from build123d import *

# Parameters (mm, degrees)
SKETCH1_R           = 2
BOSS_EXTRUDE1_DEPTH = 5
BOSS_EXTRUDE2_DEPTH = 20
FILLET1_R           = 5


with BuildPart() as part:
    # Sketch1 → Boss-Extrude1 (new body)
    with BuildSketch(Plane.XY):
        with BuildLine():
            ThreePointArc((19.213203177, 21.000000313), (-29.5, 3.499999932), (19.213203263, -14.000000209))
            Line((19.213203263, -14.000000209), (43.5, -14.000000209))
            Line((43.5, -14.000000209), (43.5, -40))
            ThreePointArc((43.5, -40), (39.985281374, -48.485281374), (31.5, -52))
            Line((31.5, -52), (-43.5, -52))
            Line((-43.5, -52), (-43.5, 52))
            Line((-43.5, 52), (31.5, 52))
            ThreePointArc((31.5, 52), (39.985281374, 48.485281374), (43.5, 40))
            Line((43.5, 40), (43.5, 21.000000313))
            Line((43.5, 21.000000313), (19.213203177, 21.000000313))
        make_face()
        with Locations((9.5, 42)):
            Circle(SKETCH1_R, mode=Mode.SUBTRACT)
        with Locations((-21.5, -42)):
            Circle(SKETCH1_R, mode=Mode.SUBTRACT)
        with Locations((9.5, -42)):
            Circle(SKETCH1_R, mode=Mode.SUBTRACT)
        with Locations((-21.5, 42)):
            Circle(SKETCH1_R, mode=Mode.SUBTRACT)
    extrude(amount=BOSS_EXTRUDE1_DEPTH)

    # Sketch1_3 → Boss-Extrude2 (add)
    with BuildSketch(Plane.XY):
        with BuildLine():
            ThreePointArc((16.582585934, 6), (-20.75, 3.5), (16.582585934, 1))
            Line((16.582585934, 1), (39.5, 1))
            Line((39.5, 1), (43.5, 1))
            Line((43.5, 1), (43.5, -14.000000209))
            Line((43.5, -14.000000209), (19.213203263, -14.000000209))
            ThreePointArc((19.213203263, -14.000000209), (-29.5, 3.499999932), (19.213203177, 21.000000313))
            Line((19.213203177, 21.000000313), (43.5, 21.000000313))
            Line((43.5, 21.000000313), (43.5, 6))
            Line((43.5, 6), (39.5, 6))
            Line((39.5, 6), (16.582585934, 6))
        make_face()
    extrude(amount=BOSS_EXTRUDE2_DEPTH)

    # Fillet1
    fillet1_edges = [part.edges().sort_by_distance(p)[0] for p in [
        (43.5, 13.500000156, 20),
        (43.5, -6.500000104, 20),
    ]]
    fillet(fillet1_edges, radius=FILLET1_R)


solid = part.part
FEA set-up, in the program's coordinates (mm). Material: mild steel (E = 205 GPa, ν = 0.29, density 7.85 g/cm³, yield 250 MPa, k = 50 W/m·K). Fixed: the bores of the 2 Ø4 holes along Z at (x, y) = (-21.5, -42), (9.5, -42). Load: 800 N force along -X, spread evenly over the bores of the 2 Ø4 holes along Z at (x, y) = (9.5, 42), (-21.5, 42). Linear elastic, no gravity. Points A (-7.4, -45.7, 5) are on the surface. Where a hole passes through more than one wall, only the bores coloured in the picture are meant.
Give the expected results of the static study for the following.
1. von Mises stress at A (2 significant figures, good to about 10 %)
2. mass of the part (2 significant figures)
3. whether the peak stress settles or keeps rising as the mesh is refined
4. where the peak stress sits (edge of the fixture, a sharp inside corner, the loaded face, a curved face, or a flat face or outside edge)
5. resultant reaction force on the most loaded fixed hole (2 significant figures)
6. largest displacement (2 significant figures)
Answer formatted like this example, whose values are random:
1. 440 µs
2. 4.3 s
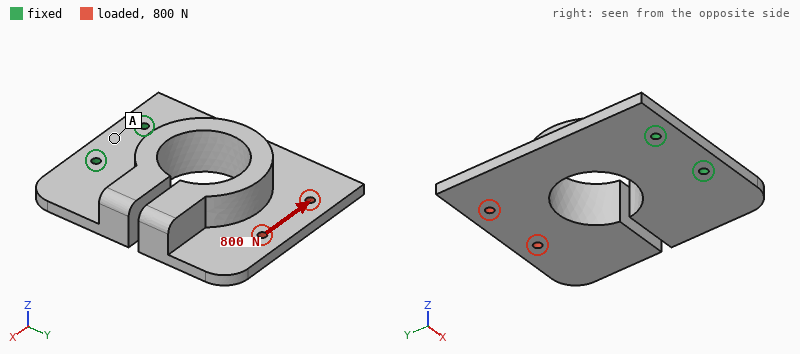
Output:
1. 8.0 MPa
2. 520 g
3. keeps rising
4. edge of the fixture
5. 2.2 kN
6. 0.11 mm
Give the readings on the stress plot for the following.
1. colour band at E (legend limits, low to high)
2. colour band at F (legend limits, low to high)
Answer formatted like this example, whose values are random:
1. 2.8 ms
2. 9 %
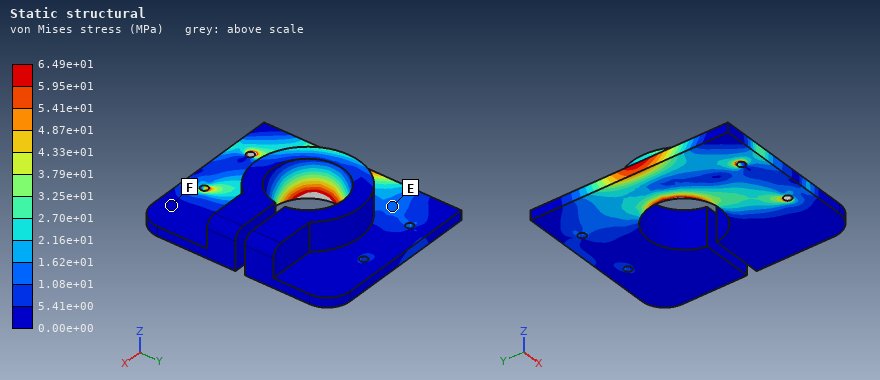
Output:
1. 1.08e+01 to 1.62e+01 MPa
2. 0.00e+00 to 5.41e+00 MPa
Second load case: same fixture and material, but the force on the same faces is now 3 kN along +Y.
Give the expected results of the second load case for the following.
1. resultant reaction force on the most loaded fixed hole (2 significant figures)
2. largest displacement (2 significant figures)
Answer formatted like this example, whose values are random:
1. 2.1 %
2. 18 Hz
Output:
1. 1.7 kN
2. 0.21 mm
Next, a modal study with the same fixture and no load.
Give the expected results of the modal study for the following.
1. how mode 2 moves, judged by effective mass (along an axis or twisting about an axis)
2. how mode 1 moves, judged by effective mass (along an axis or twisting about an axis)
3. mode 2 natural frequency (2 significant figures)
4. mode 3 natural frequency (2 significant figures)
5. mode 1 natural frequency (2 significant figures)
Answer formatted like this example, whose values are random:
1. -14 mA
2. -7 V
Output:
1. twisting about Y
2. along Z
3. 950 Hz
4. 1100 Hz
5. 350 Hz
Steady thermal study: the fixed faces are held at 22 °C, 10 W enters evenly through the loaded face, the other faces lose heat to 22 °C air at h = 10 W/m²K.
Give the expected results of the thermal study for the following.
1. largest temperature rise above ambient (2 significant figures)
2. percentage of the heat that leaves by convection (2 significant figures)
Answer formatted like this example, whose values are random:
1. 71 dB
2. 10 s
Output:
1. 48 K
2. 48 %
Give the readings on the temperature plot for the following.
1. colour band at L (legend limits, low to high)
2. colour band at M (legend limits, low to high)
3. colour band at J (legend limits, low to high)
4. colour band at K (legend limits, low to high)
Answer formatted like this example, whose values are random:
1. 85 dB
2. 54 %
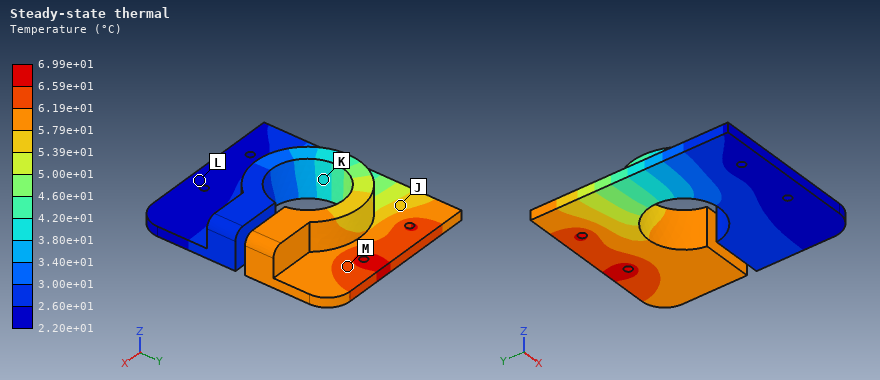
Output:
1. 2.20e+01 to 2.60e+01 °C
2. 6.19e+01 to 6.59e+01 °C
3. 5.39e+01 to 5.79e+01 °C
4. 3.80e+01 to 4.20e+01 °C
